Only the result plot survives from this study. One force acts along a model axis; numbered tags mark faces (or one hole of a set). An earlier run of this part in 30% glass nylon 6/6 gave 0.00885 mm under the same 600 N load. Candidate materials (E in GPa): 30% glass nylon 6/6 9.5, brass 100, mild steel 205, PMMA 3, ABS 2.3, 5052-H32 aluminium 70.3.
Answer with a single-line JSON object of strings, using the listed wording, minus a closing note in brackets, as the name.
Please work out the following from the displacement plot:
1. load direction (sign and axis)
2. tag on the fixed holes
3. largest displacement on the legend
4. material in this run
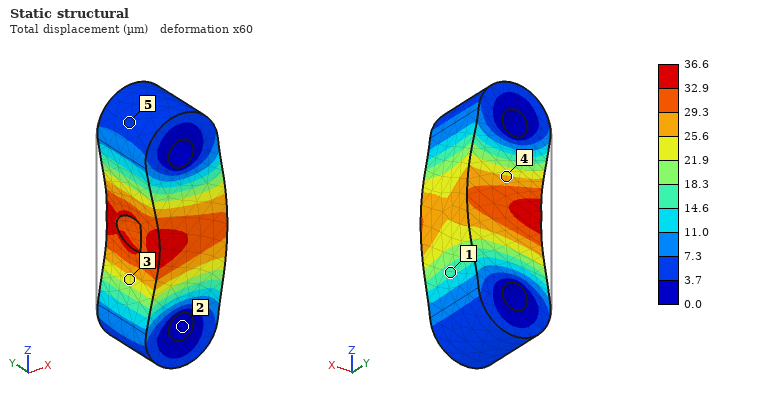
{"load direction": "+X", "tag on the fixed holes": "2", "largest displacement on the legend": "36.6 µm", "material in this run": "ABS"}
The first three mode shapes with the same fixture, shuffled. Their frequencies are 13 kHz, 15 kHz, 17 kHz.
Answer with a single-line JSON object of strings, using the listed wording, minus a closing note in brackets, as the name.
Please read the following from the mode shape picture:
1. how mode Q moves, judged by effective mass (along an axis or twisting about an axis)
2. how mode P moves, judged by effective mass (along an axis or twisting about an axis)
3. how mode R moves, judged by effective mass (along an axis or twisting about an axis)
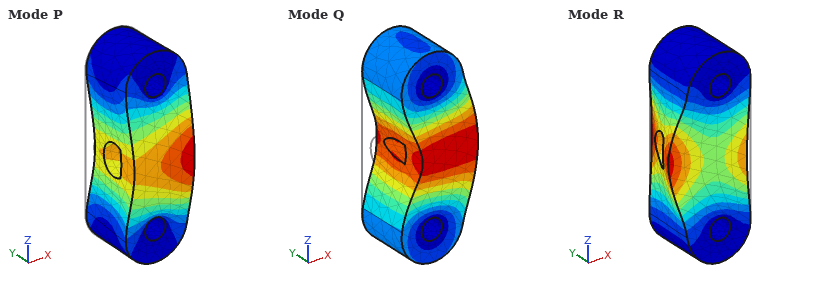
{"how mode Q moves, judged by effective mass": "along X", "how mode P moves, judged by effective mass": "along Y", "how mode R moves, judged by effective mass": "twisting about Z"}
